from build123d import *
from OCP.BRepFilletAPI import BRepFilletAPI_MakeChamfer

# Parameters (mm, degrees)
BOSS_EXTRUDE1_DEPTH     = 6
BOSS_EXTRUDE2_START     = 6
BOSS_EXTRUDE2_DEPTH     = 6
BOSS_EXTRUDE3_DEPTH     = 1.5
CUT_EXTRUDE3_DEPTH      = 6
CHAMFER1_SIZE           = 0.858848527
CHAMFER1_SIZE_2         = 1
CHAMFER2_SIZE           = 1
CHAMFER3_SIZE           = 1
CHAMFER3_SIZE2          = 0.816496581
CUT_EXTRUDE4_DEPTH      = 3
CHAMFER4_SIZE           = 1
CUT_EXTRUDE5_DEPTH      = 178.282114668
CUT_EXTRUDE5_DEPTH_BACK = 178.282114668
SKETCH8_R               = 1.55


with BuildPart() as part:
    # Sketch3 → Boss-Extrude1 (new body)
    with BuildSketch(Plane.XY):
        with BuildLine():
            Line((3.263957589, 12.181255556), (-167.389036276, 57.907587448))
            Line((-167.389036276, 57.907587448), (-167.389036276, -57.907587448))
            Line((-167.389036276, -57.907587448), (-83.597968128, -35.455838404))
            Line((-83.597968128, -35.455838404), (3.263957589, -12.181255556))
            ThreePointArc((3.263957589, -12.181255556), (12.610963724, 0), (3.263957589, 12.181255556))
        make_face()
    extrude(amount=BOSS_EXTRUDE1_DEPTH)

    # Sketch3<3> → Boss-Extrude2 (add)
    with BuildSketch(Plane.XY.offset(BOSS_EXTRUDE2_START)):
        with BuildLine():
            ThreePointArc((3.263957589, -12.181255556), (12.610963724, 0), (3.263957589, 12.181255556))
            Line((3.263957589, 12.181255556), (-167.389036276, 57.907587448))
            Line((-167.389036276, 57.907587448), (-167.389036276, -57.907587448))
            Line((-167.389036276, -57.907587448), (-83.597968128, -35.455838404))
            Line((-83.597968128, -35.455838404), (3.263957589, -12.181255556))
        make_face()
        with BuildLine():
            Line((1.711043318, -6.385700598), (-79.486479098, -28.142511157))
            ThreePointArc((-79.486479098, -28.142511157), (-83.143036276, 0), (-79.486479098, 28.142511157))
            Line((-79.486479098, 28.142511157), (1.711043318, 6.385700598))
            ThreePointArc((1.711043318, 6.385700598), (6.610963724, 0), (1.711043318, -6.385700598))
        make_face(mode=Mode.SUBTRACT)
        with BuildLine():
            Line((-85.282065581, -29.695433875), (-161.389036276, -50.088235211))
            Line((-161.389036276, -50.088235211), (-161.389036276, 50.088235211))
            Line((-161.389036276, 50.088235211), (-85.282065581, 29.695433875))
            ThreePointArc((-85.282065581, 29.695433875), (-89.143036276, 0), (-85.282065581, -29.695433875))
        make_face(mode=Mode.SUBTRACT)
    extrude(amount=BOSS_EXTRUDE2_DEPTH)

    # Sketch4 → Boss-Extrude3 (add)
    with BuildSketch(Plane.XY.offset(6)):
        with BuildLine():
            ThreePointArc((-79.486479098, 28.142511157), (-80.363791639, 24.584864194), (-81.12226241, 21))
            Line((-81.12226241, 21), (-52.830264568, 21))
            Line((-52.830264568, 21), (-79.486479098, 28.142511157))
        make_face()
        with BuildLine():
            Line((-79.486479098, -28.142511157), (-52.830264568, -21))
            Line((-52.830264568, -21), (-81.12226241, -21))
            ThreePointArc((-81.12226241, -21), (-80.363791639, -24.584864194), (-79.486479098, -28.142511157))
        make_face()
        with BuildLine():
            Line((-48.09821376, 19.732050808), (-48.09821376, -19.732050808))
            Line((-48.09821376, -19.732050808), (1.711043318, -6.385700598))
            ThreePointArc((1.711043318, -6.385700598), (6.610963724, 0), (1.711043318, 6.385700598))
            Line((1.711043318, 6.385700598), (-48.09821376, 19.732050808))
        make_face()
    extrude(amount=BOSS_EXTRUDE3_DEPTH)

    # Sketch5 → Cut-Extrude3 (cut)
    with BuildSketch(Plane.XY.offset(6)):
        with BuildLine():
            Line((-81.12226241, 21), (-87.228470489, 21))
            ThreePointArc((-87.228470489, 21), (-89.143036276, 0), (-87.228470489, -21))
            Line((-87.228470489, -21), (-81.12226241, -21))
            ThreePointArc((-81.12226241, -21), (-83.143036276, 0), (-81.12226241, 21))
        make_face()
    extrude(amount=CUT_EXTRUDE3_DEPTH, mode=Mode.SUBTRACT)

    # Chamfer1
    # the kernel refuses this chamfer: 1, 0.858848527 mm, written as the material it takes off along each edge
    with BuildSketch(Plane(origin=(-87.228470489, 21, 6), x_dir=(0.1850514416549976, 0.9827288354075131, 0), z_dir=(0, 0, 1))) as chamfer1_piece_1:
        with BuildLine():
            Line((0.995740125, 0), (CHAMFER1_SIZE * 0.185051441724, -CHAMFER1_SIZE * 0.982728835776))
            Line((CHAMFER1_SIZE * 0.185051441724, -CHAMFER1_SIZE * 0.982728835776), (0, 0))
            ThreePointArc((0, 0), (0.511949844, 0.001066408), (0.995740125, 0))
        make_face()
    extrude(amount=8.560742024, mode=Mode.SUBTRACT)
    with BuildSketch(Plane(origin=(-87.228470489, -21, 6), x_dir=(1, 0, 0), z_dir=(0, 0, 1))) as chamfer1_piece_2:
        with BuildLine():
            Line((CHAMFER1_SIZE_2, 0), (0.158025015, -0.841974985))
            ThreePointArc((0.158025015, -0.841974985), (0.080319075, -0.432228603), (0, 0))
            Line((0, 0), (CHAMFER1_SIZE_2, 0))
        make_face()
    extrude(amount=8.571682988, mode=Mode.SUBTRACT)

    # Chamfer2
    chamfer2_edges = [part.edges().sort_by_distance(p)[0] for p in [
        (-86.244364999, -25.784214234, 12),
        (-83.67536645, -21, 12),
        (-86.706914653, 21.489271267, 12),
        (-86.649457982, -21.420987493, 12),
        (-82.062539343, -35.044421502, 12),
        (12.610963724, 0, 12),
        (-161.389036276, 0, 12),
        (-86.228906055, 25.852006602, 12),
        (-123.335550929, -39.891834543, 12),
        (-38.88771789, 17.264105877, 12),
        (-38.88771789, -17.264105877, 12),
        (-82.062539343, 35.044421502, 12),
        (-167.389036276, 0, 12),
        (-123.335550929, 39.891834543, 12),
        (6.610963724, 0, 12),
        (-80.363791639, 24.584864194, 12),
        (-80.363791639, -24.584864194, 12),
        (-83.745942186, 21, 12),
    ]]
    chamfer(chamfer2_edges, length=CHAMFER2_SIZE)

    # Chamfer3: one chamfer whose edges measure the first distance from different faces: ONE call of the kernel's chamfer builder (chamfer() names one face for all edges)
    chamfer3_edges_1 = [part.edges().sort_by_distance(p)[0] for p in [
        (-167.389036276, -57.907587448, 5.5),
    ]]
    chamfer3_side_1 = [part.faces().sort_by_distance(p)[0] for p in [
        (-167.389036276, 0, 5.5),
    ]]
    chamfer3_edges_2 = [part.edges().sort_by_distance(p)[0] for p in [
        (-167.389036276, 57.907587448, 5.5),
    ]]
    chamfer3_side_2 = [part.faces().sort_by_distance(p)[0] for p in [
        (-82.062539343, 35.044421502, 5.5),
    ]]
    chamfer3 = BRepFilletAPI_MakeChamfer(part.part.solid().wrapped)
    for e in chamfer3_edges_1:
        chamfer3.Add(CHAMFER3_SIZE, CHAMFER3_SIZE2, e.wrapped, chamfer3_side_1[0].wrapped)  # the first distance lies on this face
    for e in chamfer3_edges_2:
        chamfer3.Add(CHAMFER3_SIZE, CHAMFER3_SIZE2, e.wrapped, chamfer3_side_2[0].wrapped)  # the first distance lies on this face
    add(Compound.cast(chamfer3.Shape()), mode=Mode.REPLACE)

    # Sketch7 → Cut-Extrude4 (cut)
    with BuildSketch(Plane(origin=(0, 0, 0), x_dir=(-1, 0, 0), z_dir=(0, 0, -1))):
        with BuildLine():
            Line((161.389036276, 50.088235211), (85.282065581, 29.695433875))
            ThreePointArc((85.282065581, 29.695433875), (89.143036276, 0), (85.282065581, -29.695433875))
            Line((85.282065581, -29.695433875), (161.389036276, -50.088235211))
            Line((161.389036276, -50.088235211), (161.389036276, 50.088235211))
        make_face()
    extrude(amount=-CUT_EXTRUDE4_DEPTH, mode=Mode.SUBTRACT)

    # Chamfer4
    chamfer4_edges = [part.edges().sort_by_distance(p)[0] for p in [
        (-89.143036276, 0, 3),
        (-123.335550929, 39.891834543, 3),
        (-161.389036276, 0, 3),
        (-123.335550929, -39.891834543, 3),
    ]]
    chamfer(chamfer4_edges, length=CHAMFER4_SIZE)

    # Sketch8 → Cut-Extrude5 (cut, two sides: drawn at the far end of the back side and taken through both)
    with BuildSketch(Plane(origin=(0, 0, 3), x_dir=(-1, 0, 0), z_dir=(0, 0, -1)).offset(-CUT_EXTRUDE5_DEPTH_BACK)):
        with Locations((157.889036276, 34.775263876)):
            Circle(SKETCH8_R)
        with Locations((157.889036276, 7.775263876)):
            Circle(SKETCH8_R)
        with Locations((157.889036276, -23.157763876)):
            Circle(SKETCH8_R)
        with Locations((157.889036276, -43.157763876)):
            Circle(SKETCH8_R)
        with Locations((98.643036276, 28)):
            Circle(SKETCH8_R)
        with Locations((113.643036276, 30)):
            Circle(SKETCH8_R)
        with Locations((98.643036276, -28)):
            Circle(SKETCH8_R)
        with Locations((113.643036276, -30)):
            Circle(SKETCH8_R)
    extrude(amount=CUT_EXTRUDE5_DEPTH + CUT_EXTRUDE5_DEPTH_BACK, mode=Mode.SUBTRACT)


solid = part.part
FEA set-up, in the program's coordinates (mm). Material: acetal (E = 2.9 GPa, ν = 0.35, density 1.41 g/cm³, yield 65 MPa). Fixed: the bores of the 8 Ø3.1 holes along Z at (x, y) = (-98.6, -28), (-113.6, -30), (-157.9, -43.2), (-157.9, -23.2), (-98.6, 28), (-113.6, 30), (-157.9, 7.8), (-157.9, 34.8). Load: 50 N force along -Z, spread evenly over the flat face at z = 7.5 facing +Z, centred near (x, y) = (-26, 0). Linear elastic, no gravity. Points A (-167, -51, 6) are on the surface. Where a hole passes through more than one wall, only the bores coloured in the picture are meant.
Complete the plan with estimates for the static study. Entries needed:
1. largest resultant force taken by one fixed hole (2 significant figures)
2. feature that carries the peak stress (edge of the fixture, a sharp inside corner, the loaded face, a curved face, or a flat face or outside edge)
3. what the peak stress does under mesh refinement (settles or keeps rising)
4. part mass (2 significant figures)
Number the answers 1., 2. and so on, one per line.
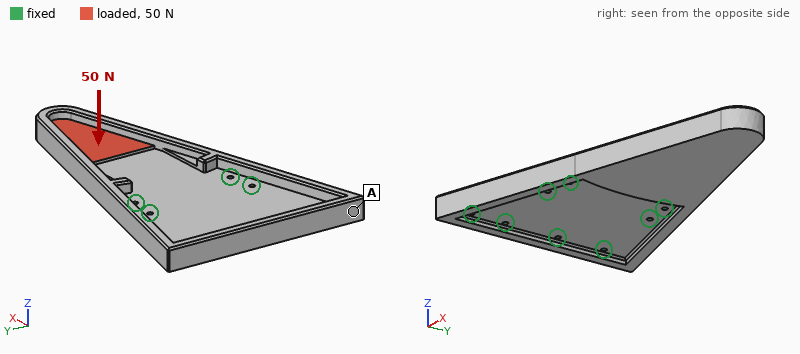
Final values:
1. 95 N
2. edge of the fixture
3. keeps rising
4. 110 g
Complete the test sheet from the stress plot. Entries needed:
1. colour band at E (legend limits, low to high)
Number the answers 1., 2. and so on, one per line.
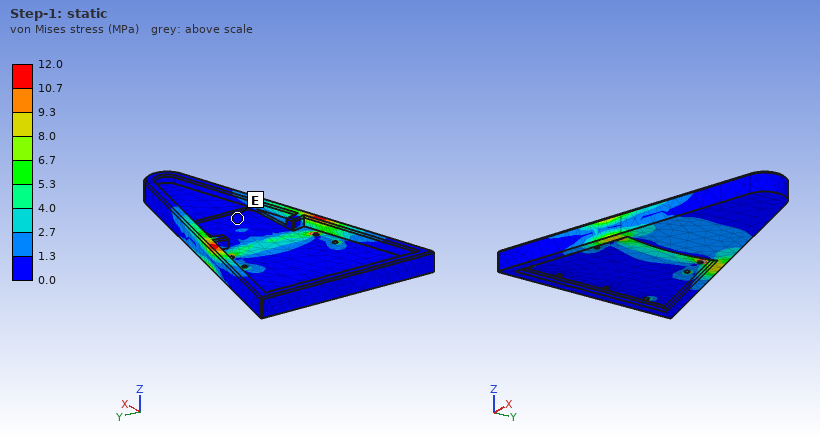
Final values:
1. 0.0 to 1.3 MPa
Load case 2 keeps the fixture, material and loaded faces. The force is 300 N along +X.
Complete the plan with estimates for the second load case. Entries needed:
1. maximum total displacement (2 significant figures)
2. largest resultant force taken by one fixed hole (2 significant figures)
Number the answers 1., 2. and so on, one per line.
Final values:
1. 0.83 mm
2. 82 N
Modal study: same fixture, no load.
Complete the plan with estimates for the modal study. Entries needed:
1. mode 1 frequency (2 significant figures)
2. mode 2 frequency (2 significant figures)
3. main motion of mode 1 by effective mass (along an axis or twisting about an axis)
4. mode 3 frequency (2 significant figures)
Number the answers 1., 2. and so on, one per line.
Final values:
1. 150 Hz
2. 760 Hz
3. along Z
4. 920 Hz
